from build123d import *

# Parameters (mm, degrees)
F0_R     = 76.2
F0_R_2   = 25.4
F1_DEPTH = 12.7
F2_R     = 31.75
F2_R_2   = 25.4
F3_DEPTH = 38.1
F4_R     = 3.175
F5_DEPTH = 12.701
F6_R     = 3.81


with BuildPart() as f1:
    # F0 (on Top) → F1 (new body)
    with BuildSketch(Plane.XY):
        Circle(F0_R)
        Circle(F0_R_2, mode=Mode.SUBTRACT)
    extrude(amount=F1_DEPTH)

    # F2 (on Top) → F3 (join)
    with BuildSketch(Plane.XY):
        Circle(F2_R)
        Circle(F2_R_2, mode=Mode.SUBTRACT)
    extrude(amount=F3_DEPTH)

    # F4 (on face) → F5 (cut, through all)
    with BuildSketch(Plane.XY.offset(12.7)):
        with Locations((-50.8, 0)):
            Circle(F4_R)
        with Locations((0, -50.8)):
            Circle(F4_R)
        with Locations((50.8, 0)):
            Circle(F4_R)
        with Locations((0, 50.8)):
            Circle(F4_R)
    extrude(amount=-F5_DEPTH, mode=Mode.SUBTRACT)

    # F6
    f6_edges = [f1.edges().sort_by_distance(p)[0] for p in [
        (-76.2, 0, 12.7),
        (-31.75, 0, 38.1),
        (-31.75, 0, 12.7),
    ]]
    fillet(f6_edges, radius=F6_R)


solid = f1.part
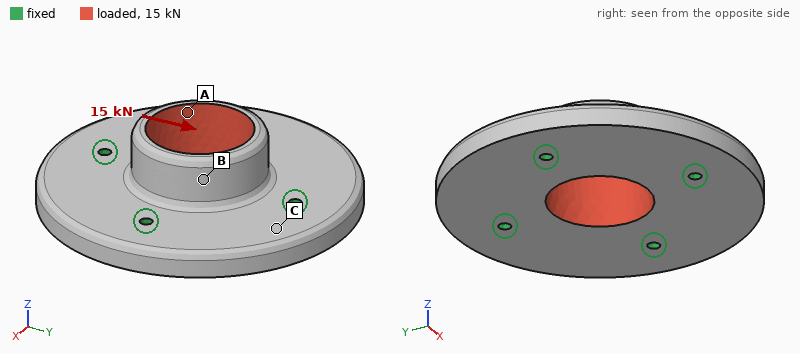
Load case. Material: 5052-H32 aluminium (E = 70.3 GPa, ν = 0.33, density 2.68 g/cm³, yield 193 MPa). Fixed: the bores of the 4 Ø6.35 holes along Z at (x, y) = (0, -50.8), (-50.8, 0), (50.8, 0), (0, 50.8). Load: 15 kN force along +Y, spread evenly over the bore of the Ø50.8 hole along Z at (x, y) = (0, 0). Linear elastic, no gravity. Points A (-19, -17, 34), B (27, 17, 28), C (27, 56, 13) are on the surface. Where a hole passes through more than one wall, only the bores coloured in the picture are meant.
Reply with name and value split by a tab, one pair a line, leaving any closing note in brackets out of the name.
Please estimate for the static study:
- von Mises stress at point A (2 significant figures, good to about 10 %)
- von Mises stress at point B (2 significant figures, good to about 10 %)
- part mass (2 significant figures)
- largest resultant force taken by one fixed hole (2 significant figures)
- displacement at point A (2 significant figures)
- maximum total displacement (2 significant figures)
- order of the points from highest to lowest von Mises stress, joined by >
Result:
von Mises stress at point A	10 MPa
von Mises stress at point B	8.0 MPa
part mass	620 g
largest resultant force taken by one fixed hole	4.6 kN
displacement at point A	21 µm
maximum total displacement	25 µm
order of the points from highest to lowest von Mises stress, joined by >	A > B > C
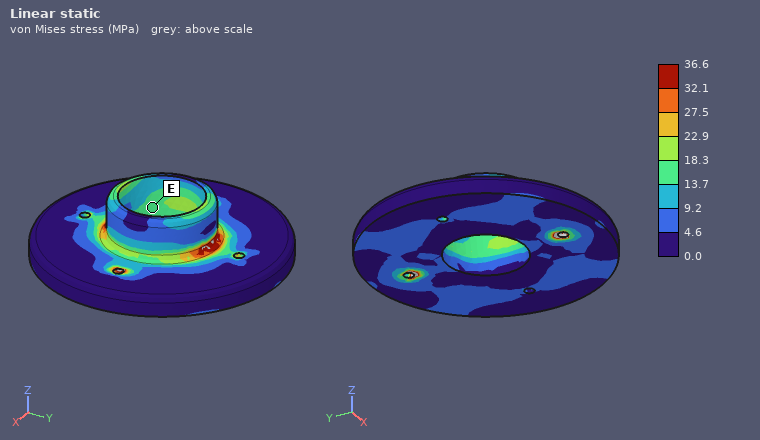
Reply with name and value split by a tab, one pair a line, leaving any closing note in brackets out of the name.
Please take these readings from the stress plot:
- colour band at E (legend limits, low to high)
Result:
colour band at E	13.7 to 18.3 MPa
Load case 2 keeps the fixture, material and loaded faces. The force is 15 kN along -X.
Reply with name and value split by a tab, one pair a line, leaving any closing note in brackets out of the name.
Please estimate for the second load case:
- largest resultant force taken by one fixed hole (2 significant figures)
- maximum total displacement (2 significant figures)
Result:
largest resultant force taken by one fixed hole	4.6 kN
maximum total displacement	25 µm
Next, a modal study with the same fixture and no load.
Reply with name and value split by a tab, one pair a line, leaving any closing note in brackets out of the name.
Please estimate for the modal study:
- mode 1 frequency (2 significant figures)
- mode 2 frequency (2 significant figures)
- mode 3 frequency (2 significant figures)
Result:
mode 1 frequency	5000 Hz
mode 2 frequency	5800 Hz
mode 3 frequency	5800 Hz
